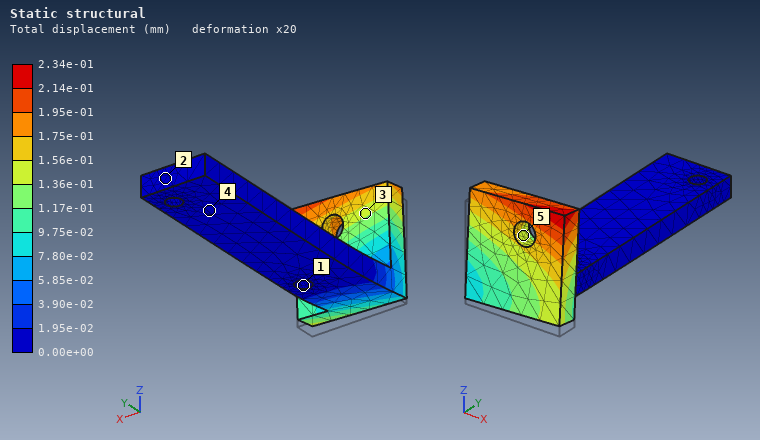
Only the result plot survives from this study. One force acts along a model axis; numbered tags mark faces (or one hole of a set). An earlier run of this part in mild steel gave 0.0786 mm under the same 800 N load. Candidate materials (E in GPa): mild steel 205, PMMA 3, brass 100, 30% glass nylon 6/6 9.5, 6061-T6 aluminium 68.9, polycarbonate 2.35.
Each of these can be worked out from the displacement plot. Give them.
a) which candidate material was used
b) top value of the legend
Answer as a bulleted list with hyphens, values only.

- 6061-T6 aluminium
- 2.34e-01 mm
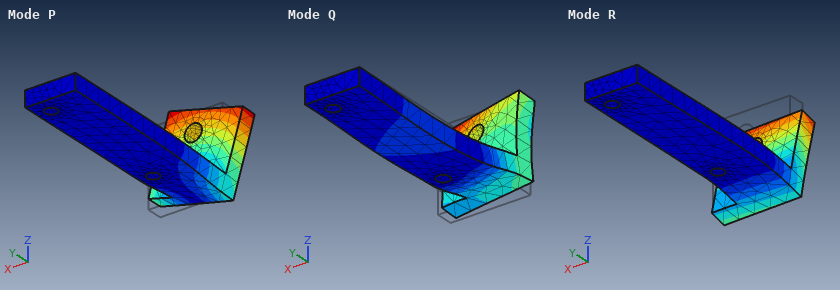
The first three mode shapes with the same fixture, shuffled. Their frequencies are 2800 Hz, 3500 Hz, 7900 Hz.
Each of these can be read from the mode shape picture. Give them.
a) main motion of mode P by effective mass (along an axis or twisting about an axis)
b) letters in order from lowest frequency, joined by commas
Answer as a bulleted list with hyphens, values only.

- along X
- R, P, Q
